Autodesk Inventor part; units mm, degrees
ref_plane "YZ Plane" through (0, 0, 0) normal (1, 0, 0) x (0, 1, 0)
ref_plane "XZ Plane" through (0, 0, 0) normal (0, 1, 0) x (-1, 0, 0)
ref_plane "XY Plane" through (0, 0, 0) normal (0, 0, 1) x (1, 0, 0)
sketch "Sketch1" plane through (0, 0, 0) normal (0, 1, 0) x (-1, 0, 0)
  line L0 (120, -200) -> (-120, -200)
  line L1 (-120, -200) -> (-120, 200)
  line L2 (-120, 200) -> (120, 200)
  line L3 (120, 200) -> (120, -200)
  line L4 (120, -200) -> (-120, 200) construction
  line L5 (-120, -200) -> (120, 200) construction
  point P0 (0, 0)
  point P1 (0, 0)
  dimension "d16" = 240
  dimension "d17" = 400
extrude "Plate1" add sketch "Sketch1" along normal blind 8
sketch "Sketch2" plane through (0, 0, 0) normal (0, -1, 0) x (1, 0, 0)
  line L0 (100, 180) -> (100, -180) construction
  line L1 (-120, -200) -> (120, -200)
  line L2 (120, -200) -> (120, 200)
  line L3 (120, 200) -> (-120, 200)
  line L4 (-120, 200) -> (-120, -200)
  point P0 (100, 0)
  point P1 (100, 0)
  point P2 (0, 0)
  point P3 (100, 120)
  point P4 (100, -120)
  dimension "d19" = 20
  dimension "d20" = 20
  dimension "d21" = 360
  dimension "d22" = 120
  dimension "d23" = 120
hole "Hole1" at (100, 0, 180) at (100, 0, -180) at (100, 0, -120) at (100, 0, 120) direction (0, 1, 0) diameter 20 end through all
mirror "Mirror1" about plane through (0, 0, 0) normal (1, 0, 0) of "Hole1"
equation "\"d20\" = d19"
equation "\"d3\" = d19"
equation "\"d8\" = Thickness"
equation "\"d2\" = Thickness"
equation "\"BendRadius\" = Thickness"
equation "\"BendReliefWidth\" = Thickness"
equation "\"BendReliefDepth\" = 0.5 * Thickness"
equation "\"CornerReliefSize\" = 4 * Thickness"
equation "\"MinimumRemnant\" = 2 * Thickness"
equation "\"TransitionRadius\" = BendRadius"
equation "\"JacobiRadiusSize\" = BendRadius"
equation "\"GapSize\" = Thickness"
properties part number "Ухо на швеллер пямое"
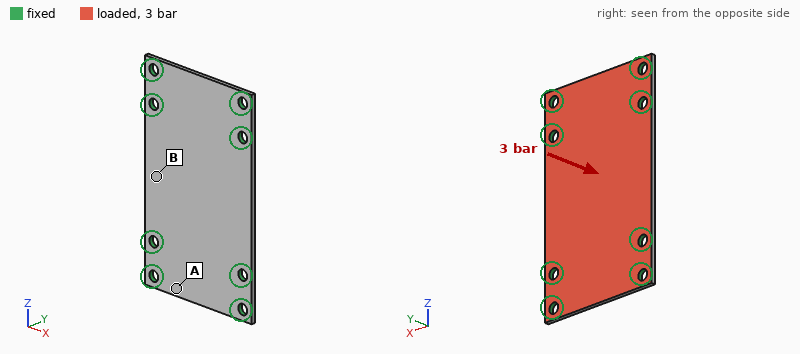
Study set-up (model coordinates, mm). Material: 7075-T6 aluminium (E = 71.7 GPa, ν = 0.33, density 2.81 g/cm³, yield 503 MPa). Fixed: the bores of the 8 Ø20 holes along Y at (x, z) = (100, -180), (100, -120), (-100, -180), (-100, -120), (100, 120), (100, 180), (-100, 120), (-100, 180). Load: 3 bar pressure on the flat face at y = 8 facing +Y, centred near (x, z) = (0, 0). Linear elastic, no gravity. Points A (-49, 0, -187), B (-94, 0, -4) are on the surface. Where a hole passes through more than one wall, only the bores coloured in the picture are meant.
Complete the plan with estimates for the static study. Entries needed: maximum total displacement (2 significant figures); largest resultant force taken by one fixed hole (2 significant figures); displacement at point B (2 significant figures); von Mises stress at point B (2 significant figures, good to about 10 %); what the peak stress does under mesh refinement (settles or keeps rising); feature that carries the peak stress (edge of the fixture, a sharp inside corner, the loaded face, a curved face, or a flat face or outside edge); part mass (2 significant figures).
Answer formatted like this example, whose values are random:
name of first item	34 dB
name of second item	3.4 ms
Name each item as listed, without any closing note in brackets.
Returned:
maximum total displacement	1.3 mm
largest resultant force taken by one fixed hole	5.9 kN
displacement at point B	0.92 mm
von Mises stress at point B	71 MPa
what the peak stress does under mesh refinement	keeps rising
feature that carries the peak stress	edge of the fixture
part mass	2.1 kg
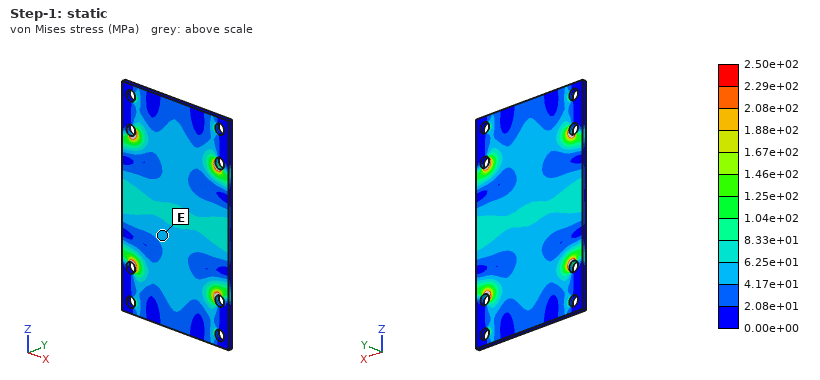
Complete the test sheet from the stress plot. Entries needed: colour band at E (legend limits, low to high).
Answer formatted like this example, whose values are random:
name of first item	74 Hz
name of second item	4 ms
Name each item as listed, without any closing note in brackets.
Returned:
colour band at E	4.17e+01 to 6.25e+01 MPa
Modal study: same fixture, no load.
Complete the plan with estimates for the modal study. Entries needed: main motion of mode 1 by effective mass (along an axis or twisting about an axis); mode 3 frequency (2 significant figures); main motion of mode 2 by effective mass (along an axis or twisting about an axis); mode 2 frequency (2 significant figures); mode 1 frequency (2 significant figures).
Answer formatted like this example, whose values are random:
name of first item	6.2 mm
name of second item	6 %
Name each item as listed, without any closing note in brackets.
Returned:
main motion of mode 1 by effective mass	along Y
mode 3 frequency	1200 Hz
main motion of mode 2 by effective mass	twisting about Z
mode 2 frequency	940 Hz
mode 1 frequency	630 Hz
